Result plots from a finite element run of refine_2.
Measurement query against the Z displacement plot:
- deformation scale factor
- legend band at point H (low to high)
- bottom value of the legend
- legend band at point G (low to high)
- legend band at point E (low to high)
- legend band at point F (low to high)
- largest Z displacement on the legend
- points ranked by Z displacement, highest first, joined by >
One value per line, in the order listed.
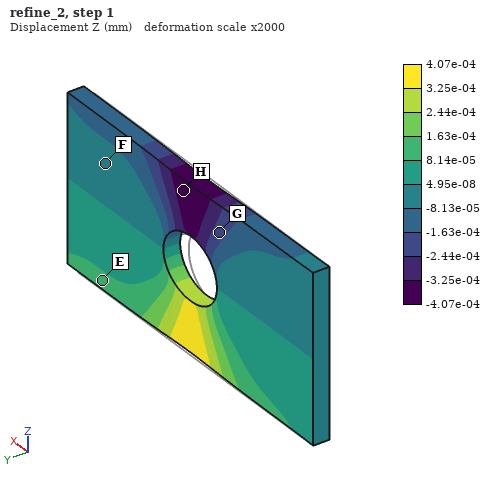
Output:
2000
-4.07e-04 to -3.25e-04 mm
-4.07e-04 mm
-2.44e-04 to -1.63e-04 mm
8.14e-05 to 1.63e-04 mm
-8.13e-05 to 4.95e-08 mm
4.07e-04 mm
E > F > G > H
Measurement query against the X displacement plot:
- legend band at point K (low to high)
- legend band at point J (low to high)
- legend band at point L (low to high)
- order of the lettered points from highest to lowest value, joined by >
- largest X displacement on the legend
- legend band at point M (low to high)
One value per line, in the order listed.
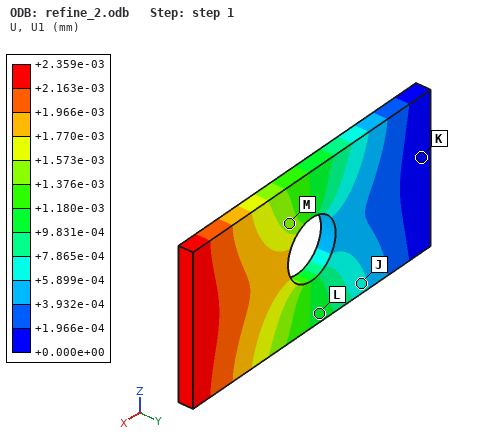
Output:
+0.000e+00 to +1.966e-04 mm
+5.899e-04 to +7.865e-04 mm
+9.831e-04 to +1.180e-03 mm
M > L > J > K
+2.359e-03 mm
+1.376e-03 to +1.573e-03 mm
